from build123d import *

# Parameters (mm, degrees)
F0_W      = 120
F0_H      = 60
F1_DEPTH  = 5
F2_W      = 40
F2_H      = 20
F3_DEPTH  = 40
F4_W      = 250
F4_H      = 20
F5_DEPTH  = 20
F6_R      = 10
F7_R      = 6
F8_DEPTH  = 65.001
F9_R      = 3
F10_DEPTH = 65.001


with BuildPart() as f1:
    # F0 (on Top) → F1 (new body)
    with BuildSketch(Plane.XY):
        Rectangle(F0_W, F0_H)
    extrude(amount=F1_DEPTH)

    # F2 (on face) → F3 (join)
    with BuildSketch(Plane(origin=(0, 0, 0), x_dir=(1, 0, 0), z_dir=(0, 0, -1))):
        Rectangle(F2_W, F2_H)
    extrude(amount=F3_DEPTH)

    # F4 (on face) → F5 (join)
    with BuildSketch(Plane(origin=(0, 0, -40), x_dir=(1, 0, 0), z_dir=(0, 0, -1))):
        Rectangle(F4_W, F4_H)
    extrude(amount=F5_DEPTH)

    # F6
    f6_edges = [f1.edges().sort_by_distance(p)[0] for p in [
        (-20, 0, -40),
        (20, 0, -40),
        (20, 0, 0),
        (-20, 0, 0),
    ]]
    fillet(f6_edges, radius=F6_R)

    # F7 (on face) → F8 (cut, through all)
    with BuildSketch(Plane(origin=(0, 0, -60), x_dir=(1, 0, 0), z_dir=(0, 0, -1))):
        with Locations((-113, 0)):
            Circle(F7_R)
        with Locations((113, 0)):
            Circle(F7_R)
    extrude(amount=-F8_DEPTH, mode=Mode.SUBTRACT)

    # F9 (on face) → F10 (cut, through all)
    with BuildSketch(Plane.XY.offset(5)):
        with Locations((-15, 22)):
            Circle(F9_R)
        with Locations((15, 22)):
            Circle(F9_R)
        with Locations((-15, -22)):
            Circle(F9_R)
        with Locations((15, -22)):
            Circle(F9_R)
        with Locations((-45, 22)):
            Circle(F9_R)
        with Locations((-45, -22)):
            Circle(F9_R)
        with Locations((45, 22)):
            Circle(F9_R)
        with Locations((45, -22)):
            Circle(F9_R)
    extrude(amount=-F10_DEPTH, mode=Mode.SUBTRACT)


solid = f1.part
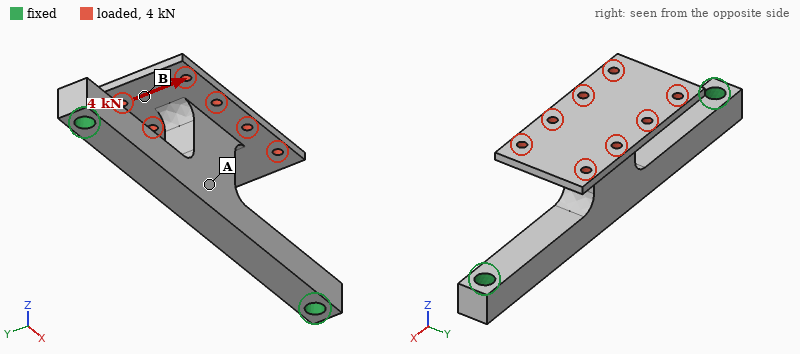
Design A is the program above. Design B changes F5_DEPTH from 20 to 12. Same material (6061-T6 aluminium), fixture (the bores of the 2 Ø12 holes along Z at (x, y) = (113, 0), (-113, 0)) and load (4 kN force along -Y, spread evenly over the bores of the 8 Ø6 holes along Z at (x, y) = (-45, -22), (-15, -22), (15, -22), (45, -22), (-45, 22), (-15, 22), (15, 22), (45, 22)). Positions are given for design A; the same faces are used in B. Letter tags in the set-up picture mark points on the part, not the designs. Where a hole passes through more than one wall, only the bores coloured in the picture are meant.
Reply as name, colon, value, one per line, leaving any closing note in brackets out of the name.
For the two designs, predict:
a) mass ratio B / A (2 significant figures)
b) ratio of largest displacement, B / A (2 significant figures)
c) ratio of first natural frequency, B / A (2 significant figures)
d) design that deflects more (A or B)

mass ratio B / A: 0.77
ratio of largest displacement, B / A: 2.2
ratio of first natural frequency, B / A: 0.69
design that deflects more: B
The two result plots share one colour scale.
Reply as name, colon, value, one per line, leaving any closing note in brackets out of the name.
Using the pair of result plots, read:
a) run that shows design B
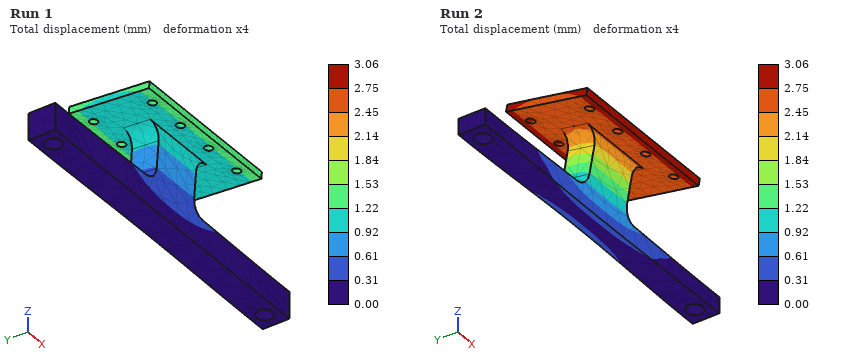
run that shows design B: Run 2
